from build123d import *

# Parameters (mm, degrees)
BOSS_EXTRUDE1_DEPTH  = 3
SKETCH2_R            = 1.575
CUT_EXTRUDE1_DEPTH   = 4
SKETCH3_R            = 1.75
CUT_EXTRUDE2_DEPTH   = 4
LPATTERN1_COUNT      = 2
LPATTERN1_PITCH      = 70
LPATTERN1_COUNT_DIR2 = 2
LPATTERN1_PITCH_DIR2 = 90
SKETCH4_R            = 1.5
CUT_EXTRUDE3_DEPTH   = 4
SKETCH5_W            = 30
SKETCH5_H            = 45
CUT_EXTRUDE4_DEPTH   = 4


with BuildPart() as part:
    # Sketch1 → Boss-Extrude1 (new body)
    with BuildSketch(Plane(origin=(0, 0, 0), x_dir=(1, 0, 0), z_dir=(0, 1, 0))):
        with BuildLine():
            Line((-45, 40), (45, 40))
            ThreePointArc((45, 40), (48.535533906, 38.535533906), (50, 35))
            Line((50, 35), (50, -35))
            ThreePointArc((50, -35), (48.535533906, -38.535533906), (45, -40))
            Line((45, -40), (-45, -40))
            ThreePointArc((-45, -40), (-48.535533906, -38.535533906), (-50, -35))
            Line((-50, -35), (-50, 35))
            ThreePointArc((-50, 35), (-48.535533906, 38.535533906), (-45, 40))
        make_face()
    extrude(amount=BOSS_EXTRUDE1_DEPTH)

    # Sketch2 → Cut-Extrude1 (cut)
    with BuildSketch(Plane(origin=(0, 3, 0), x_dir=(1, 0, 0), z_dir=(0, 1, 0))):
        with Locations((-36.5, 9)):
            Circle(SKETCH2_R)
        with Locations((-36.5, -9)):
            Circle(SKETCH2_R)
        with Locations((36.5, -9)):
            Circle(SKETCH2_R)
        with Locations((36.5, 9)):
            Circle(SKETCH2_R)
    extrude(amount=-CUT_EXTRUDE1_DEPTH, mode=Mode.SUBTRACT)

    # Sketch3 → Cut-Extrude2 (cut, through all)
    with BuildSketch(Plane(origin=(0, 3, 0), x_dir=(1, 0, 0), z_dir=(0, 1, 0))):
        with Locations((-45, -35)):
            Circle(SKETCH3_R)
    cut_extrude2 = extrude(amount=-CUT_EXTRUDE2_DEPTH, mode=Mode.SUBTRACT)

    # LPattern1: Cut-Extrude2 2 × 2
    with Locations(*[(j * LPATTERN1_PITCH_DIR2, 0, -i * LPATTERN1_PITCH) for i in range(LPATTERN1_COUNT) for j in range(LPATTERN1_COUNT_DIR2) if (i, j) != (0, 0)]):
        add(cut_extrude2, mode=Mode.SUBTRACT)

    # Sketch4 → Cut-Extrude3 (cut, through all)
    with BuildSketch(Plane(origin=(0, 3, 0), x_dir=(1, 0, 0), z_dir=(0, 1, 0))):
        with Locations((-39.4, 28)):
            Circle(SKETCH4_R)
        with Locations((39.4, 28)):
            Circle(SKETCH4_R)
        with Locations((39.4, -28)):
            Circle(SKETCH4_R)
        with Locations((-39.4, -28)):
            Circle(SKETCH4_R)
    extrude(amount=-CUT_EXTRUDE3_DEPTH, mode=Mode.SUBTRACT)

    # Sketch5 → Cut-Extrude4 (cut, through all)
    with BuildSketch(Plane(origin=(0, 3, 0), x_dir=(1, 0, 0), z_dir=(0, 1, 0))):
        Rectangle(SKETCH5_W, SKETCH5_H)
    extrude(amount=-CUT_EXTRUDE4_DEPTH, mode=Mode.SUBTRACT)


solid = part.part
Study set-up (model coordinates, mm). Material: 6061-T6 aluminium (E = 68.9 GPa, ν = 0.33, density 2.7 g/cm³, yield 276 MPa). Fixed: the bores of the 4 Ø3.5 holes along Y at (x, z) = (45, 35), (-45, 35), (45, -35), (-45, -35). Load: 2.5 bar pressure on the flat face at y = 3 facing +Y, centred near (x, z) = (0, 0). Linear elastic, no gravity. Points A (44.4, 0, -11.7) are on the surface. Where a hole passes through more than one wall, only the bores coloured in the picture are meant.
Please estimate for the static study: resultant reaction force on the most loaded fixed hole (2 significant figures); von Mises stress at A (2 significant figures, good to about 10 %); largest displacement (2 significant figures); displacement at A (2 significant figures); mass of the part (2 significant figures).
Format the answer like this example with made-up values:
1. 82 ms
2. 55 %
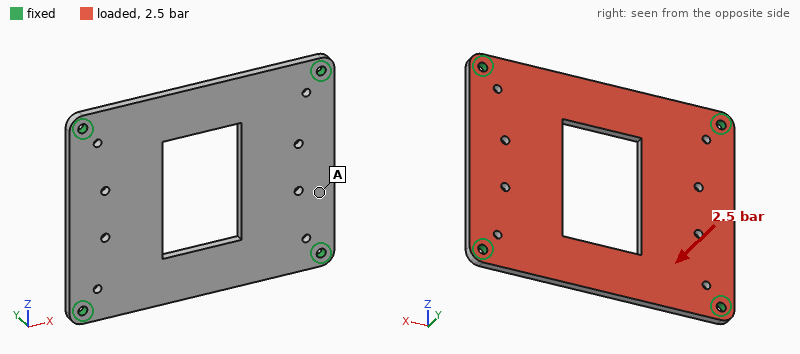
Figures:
1. 410 N
2. 35 MPa
3. 0.53 mm
4. 0.12 mm
5. 53 g
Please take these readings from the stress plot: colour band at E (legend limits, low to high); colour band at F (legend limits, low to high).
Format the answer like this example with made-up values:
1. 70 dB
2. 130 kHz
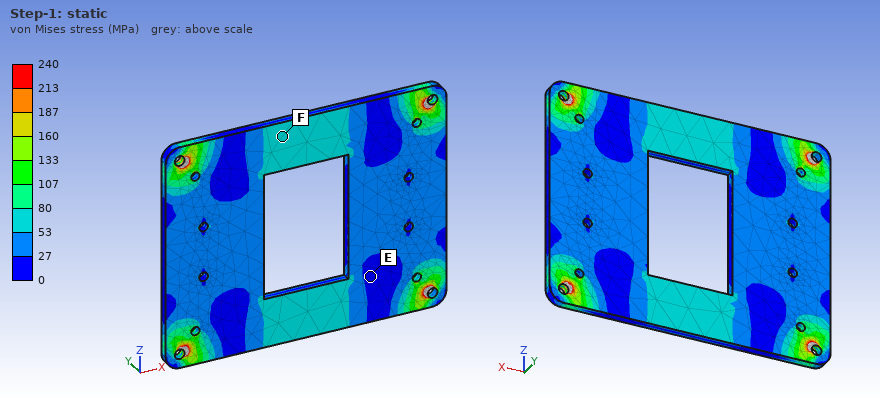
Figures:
1. 0 to 27 MPa
2. 53 to 80 MPa
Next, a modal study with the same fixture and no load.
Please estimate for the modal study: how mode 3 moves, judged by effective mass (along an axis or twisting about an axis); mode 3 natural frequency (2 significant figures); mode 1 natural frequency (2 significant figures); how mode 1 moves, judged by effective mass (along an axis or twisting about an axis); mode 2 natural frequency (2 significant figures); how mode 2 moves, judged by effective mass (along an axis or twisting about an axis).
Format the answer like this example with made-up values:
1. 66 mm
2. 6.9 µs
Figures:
1. twisting about Z
2. 2600 Hz
3. 1500 Hz
4. along Y
5. 2300 Hz
6. twisting about X
